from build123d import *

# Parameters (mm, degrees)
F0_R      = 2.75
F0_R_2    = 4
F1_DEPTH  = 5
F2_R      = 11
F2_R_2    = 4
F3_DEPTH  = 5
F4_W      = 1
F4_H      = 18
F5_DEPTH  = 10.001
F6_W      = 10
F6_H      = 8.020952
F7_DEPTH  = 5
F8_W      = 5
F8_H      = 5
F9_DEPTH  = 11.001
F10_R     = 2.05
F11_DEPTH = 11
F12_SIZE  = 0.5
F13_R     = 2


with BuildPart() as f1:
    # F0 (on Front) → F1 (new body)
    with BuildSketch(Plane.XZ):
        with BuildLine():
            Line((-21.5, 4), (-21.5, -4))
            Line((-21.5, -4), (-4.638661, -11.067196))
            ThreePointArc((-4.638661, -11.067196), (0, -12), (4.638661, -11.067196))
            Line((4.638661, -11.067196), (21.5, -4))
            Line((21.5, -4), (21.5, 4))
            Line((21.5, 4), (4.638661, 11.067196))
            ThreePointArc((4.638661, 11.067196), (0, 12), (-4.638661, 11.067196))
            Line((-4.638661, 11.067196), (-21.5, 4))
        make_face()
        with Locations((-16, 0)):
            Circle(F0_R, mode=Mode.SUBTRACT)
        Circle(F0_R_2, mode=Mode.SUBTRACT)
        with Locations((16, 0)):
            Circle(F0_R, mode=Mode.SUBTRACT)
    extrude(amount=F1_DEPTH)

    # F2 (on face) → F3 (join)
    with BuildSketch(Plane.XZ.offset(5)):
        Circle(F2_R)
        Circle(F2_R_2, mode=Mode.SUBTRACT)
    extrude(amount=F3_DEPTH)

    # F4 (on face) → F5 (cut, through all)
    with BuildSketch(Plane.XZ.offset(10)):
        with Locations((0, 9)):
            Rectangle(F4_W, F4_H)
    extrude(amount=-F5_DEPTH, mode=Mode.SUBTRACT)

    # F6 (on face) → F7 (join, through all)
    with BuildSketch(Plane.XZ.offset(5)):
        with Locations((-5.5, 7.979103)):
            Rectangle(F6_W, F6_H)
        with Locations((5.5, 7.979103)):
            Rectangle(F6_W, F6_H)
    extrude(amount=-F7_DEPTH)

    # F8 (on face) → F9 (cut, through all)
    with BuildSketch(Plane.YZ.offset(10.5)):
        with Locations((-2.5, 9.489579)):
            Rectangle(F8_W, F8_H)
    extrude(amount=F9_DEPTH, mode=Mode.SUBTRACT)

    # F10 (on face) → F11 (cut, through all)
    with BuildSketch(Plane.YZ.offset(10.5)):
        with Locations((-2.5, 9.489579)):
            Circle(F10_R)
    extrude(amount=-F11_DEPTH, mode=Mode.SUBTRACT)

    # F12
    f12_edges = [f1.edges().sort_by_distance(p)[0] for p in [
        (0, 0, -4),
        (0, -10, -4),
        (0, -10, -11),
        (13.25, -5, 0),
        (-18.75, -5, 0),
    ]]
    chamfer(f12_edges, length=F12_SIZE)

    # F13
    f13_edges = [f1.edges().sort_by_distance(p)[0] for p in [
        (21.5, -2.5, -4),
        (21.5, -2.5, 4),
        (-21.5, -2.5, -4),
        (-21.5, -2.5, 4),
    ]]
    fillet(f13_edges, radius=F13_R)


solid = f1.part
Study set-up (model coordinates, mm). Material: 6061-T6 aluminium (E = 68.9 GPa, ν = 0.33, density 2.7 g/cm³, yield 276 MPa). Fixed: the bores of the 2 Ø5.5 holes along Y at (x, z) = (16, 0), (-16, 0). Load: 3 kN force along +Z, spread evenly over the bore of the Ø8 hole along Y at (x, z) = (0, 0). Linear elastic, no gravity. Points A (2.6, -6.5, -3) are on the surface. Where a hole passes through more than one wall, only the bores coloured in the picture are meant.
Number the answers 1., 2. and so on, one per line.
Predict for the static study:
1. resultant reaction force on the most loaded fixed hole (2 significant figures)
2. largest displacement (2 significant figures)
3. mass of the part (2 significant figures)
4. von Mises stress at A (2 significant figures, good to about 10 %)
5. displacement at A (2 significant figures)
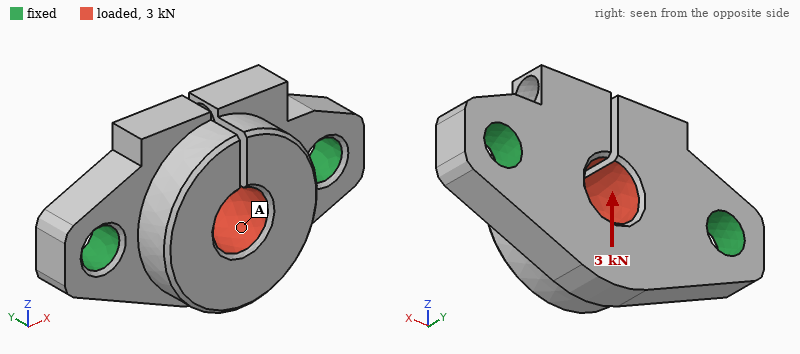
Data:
1. 1.9 kN
2. 37 µm
3. 13 g
4. 21 MPa
5. 21 µm
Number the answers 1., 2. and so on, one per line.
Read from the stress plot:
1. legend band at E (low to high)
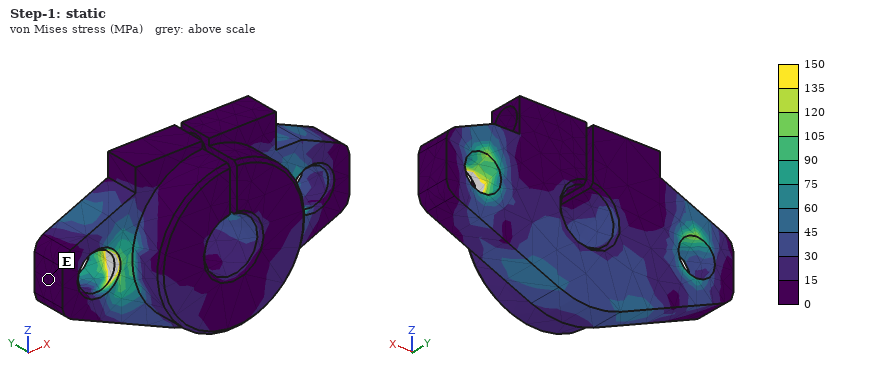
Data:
1. 0 to 15 MPa
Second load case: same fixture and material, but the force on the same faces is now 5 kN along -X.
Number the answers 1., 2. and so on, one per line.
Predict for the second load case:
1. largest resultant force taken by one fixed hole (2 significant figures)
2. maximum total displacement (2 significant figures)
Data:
1. 2.5 kN
2. 21 µm
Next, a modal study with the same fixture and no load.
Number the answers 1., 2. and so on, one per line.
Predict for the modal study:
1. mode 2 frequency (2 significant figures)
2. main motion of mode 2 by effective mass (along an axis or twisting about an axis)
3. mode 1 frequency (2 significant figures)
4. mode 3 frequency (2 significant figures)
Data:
1. 18 kHz
2. along Y
3. 15 kHz
4. 19 kHz
